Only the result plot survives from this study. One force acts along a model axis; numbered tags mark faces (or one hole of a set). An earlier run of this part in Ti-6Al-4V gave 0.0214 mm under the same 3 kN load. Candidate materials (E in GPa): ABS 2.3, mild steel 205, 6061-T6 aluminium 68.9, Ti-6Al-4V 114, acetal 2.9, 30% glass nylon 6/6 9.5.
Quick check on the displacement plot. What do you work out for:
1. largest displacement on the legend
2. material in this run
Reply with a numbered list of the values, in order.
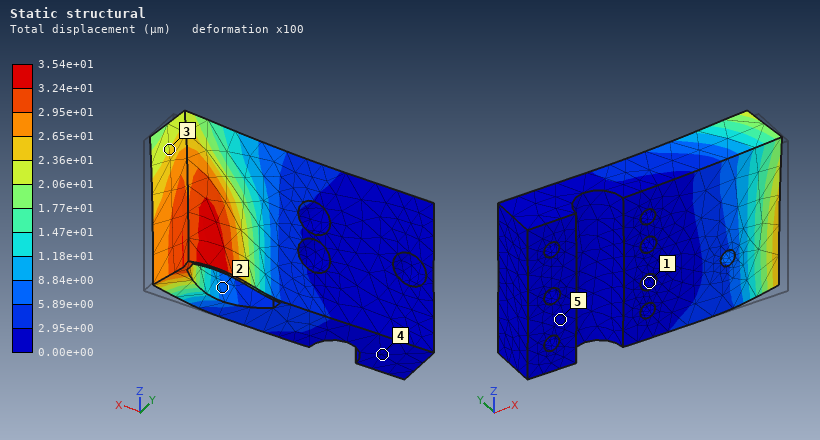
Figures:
1. 3.54e+01 µm
2. 6061-T6 aluminium
